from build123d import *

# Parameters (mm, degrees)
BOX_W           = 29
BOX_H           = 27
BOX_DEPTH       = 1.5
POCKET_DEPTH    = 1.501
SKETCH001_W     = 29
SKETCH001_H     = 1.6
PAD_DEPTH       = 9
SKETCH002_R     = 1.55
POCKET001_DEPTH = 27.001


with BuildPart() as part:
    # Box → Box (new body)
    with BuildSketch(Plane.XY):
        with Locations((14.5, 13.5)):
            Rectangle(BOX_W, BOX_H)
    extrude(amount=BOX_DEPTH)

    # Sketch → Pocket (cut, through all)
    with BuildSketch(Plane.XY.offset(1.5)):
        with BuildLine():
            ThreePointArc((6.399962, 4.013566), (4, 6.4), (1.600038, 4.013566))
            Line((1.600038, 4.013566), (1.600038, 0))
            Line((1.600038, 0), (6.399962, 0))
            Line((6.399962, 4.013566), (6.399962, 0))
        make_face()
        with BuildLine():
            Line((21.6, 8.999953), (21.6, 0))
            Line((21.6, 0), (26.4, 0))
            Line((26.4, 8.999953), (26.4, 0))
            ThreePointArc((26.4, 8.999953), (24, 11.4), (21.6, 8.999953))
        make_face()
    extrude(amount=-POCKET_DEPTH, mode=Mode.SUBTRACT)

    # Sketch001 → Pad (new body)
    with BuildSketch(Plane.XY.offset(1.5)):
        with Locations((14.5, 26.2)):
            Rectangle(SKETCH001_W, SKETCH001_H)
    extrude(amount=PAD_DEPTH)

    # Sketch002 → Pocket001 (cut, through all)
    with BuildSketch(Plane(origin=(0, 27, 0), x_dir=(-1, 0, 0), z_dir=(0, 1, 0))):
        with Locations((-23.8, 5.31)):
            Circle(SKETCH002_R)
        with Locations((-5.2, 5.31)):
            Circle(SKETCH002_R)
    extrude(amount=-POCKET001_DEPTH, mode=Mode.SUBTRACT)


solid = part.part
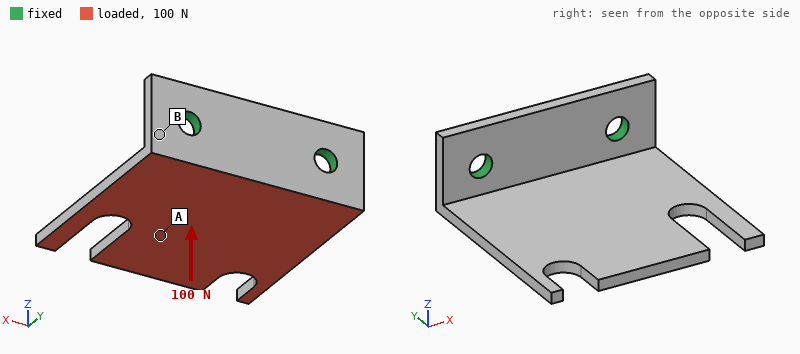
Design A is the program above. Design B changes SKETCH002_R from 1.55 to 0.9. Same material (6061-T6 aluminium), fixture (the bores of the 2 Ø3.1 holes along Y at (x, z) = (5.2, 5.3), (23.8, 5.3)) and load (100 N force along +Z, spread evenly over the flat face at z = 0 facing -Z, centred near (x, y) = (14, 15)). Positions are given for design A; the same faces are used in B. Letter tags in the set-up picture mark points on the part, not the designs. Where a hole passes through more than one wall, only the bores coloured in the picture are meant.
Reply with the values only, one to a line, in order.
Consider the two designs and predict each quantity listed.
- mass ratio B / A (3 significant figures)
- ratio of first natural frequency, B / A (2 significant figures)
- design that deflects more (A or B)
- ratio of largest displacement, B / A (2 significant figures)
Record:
1.01
0.95
B
1.1
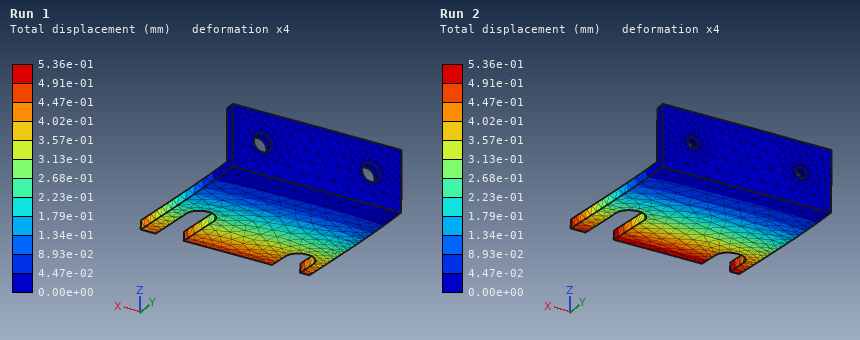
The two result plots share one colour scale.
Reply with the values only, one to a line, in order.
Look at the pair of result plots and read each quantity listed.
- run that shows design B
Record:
Run 2
